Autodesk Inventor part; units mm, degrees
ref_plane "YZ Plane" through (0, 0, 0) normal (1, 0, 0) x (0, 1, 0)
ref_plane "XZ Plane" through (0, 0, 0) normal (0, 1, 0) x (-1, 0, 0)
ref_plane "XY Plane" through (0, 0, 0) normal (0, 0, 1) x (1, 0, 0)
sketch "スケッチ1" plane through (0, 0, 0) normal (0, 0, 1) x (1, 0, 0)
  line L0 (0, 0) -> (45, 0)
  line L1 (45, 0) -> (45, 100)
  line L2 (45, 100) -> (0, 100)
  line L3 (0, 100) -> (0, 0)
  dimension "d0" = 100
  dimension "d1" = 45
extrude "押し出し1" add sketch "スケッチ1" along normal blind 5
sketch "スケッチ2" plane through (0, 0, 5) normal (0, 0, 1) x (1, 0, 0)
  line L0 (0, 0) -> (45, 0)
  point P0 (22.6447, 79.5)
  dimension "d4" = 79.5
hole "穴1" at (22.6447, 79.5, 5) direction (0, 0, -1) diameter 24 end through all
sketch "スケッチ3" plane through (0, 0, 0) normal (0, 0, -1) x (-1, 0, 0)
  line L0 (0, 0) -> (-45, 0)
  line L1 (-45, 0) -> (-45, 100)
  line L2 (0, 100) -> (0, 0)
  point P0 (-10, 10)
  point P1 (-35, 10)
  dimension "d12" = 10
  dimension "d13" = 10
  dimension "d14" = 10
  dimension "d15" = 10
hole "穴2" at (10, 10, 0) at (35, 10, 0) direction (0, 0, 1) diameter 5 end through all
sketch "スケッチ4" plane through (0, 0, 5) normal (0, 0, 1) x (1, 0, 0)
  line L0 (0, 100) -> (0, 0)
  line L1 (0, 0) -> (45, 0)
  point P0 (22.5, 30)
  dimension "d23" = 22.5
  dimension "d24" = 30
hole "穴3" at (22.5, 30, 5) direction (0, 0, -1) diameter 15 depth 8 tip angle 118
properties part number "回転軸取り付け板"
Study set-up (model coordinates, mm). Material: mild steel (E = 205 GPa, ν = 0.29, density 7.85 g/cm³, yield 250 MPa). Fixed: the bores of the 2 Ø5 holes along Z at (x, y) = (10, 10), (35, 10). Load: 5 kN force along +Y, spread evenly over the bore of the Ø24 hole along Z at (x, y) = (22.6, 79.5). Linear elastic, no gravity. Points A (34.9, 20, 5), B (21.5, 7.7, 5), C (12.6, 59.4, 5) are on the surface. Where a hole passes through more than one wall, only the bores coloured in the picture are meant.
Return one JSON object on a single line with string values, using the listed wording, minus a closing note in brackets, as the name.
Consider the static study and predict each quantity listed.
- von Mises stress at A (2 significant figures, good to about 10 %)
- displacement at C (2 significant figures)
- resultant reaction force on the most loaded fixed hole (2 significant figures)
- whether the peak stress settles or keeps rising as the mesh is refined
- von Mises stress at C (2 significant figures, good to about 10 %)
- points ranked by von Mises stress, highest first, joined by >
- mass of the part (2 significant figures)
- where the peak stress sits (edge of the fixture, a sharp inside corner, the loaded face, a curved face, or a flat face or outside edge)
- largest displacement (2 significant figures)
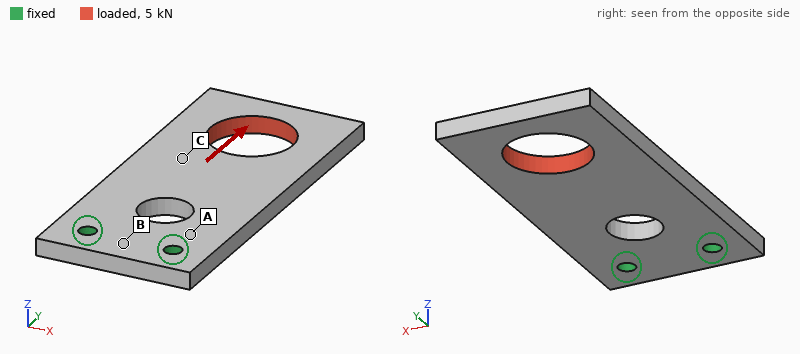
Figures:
{"von Mises stress at A": "38 MPa", "displacement at C": "7.0 µm", "resultant reaction force on the most loaded fixed hole": "2.5 kN", "whether the peak stress settles or keeps rising as the mesh is refined": "keeps rising", "von Mises stress at C": "22 MPa", "points ranked by von Mises stress, highest first, joined by >": "A > C > B", "mass of the part": "150 g", "where the peak stress sits": "edge of the fixture", "largest displacement": "16 µm"}
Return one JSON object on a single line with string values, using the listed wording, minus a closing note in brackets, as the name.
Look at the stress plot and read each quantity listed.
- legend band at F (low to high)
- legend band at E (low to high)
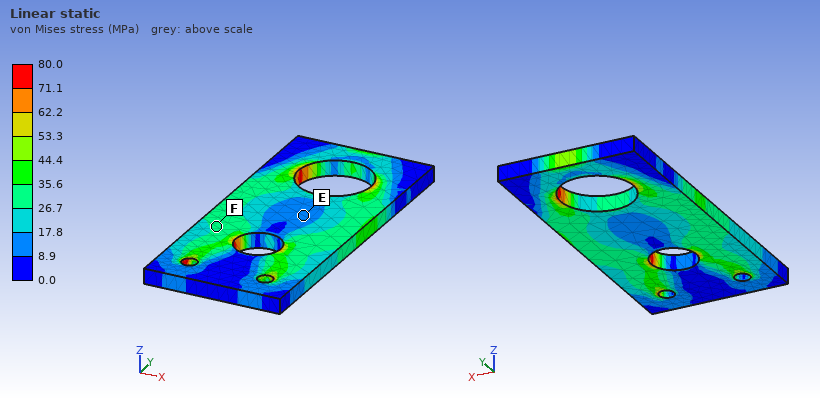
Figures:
{"legend band at F": "26.7 to 35.6 MPa", "legend band at E": "8.9 to 17.8 MPa"}
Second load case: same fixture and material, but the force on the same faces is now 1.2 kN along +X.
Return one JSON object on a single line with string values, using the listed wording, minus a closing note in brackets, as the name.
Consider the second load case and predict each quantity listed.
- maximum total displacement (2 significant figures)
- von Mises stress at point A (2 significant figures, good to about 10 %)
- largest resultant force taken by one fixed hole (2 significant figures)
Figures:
{"maximum total displacement": "46 µm", "von Mises stress at point A": "33 MPa", "largest resultant force taken by one fixed hole": "3.0 kN"}
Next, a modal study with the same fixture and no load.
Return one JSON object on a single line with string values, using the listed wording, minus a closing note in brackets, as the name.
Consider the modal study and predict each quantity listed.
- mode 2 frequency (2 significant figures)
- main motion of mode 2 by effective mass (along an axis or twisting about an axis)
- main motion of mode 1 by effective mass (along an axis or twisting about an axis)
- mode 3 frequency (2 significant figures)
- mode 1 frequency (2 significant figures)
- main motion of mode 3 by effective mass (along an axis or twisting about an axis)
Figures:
{"mode 2 frequency": "2000 Hz", "main motion of mode 2 by effective mass": "twisting about Y", "main motion of mode 1 by effective mass": "along Z", "mode 3 frequency": "2900 Hz", "mode 1 frequency": "530 Hz", "main motion of mode 3 by effective mass": "along Z"}
